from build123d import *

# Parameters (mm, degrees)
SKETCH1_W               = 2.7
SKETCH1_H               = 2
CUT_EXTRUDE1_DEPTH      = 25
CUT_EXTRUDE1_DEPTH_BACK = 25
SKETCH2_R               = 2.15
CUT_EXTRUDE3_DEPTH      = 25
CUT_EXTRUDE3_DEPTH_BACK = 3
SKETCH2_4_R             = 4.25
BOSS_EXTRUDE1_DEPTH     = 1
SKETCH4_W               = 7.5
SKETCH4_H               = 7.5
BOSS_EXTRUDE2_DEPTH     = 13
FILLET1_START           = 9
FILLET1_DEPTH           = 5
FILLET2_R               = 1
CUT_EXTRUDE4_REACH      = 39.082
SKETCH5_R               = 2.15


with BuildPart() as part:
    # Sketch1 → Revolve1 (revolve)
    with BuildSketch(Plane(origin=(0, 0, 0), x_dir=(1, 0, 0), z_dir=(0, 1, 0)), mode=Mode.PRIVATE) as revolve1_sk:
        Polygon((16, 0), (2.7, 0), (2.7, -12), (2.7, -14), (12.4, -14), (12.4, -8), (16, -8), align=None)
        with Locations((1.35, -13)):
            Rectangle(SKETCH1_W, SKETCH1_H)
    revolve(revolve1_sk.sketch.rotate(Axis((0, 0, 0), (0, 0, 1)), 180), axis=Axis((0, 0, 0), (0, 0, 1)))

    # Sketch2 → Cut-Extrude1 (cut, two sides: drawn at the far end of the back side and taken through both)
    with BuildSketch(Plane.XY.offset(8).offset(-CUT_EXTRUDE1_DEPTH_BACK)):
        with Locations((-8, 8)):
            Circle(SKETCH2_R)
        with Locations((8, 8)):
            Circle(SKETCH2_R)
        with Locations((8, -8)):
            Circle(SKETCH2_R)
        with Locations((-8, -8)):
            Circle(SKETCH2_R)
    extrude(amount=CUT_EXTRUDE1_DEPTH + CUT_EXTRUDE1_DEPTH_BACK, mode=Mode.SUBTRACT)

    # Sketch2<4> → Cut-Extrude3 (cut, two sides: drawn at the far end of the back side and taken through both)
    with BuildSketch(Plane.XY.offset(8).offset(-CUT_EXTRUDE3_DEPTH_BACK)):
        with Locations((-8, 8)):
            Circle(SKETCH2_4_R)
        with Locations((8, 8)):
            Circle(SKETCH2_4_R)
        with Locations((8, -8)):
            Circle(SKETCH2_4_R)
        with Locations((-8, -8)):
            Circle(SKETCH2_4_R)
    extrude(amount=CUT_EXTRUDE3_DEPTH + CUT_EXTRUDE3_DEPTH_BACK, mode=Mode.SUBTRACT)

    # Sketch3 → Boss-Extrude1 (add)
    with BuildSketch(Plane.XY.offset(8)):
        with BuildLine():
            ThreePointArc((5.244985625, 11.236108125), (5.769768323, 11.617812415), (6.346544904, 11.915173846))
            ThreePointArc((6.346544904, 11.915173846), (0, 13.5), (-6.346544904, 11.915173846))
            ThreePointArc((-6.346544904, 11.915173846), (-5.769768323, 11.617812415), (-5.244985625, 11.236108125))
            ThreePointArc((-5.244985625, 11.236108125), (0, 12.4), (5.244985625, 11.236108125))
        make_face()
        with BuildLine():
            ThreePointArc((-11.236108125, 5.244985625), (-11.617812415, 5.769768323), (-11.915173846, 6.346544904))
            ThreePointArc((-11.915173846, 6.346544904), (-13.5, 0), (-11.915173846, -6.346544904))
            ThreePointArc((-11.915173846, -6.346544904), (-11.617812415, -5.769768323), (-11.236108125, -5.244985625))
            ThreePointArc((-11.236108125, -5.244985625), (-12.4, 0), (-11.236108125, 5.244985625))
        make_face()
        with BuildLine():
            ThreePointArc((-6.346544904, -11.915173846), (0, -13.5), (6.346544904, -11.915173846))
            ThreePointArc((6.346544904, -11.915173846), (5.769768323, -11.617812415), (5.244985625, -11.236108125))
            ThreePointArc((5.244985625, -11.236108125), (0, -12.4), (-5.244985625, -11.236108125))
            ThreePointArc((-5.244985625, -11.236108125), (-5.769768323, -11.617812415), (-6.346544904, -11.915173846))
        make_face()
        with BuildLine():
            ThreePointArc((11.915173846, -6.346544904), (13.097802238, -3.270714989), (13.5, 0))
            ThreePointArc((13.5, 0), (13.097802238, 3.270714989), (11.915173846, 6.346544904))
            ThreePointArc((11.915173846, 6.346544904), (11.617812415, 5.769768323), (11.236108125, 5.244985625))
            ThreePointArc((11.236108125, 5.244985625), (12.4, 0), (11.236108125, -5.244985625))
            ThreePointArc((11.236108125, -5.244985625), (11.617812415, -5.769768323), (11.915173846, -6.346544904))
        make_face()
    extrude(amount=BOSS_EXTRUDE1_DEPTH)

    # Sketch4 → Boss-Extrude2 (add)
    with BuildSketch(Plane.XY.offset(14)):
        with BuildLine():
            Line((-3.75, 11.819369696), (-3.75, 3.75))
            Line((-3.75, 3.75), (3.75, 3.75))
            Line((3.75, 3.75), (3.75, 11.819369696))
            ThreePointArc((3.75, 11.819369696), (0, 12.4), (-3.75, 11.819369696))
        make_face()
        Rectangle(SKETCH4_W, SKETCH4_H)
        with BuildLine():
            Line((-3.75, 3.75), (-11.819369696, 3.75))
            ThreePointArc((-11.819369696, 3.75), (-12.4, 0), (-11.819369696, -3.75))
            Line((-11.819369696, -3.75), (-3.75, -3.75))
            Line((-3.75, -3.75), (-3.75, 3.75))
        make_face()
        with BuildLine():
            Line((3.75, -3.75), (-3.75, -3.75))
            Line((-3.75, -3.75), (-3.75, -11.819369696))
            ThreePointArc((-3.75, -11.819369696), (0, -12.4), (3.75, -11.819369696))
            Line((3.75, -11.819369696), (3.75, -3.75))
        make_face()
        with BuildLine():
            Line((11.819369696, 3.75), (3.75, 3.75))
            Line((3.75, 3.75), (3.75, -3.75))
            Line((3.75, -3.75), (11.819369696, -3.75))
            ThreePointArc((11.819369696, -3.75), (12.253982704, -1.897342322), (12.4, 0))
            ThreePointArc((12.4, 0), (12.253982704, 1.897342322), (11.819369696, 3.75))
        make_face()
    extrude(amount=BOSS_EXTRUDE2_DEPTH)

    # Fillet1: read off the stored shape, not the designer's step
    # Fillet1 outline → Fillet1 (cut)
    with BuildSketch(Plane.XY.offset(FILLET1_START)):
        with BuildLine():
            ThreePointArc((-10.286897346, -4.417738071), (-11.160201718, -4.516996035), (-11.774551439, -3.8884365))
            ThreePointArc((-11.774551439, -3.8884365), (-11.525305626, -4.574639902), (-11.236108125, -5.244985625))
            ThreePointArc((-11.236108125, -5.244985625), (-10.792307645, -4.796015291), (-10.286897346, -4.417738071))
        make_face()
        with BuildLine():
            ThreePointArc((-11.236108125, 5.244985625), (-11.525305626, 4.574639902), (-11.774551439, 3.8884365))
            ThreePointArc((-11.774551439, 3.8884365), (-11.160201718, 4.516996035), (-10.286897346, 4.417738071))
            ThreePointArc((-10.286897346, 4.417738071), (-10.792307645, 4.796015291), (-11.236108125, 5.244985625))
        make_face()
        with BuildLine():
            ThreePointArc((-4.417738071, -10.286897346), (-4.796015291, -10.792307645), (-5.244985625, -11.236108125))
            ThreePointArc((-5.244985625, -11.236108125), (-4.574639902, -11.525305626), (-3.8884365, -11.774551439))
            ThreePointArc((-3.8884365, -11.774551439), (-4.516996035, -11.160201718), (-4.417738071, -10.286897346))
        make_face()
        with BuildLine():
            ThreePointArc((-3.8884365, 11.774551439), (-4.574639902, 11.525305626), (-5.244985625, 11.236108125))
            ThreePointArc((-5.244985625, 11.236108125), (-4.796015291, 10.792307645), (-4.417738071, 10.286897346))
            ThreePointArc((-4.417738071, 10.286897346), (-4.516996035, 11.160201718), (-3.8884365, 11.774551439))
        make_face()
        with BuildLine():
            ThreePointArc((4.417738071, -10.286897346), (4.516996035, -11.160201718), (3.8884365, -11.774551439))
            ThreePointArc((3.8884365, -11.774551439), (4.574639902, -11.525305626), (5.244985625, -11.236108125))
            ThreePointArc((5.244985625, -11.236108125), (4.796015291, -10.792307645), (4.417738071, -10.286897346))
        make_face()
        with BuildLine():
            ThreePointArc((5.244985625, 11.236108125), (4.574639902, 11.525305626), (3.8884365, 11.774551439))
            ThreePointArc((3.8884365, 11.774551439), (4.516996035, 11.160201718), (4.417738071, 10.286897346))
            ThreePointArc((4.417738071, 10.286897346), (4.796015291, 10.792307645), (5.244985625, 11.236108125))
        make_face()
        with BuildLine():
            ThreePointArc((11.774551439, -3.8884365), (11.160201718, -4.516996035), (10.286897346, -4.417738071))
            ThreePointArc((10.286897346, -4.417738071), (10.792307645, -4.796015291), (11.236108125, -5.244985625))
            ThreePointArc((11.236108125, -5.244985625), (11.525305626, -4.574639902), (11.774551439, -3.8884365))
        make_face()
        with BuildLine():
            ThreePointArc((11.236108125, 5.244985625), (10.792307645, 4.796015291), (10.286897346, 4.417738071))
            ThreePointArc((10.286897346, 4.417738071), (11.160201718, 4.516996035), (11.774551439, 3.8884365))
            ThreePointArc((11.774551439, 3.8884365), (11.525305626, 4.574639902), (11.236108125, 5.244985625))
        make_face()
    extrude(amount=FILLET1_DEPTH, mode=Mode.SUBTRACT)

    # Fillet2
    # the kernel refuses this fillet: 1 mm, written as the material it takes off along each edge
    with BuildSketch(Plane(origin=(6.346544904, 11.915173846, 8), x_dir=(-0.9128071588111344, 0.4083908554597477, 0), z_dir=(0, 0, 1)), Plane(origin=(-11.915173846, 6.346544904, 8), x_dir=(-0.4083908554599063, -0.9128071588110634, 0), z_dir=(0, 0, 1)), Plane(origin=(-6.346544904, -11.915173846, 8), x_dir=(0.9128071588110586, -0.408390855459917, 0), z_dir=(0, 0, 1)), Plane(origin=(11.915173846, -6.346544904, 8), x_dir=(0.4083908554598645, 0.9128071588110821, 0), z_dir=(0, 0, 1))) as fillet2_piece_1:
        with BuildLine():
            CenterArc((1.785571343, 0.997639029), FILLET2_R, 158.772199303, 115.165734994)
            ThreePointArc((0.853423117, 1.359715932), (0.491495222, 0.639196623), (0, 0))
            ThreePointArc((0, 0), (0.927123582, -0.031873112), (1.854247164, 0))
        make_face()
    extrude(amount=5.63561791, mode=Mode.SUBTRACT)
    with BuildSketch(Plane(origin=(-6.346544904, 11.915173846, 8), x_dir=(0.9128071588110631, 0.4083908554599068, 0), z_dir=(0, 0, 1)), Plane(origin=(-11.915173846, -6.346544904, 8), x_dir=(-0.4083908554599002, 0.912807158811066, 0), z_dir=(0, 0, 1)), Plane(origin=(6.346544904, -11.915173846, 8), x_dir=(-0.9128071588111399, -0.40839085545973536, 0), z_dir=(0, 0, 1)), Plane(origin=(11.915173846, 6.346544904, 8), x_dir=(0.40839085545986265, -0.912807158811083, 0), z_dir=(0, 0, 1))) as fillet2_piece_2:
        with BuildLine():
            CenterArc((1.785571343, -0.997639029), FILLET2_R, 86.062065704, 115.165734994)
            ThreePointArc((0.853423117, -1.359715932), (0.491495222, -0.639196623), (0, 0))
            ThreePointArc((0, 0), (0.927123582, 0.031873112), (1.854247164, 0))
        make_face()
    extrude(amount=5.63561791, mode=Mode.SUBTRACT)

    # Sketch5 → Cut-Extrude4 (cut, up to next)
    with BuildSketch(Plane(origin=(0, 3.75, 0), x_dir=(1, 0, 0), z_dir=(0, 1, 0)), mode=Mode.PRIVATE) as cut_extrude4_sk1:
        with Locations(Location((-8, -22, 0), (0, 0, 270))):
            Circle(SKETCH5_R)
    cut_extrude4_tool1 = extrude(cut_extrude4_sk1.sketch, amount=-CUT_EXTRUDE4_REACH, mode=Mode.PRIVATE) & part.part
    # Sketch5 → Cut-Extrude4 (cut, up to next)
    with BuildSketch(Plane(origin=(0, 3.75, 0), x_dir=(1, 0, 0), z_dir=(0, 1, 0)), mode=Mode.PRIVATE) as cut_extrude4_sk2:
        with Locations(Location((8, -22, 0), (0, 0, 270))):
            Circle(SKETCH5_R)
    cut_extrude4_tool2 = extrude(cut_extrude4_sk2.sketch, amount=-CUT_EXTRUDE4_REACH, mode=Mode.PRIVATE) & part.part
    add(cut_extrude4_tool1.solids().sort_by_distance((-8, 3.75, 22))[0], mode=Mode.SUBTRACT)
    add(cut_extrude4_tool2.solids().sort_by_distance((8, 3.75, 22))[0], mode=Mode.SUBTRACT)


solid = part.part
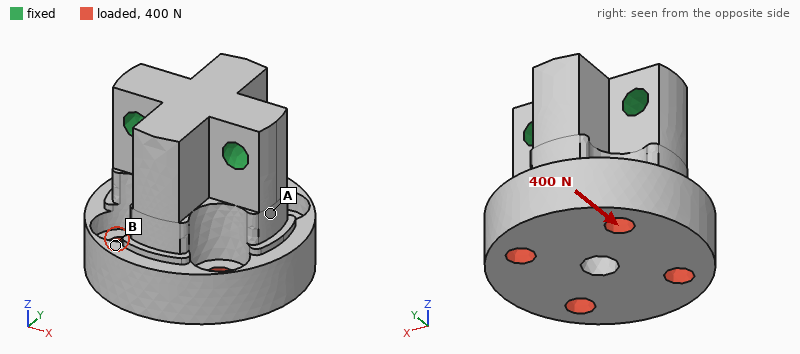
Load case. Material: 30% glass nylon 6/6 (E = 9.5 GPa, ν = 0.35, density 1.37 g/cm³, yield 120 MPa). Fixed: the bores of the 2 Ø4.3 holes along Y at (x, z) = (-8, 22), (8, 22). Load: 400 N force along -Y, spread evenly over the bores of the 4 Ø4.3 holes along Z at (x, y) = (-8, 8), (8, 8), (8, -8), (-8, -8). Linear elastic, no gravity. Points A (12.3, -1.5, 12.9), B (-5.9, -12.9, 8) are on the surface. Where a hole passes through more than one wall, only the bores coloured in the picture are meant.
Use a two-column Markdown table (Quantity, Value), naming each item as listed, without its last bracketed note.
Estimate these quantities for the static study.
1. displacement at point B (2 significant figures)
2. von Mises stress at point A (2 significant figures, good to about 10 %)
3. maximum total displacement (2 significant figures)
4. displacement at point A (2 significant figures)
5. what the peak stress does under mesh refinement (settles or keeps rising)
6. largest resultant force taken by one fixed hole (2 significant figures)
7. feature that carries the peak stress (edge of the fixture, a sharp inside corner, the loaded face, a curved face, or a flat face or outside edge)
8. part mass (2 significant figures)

| Quantity | Value |
|---|---|
| displacement at point B | 0.073 mm |
| von Mises stress at point A | 8.1 MPa |
| maximum total displacement | 0.10 mm |
| displacement at point A | 0.026 mm |
| what the peak stress does under mesh refinement | keeps rising |
| largest resultant force taken by one fixed hole | 200 N |
| feature that carries the peak stress | edge of the fixture |
| part mass | 15 g |
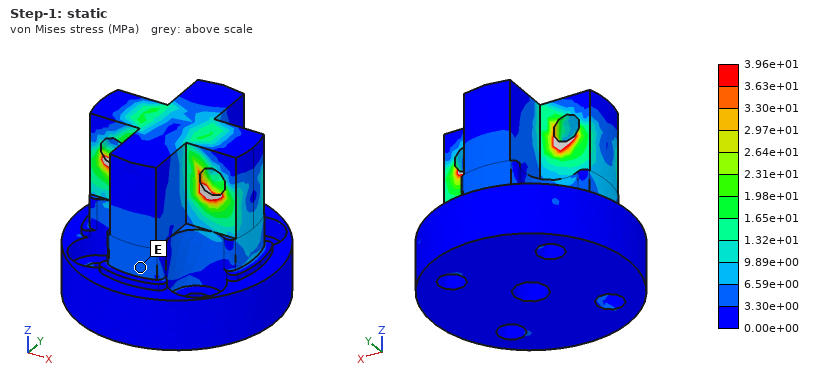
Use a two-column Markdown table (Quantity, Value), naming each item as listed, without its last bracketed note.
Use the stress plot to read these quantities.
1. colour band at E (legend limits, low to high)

| Quantity | Value |
|---|---|
| colour band at E | 3.30e+00 to 6.59e+00 MPa |
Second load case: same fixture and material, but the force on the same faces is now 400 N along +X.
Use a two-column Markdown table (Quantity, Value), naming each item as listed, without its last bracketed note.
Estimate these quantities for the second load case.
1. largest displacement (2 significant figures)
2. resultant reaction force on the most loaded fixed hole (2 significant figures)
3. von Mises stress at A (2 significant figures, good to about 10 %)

| Quantity | Value |
|---|---|
| largest displacement | 27 µm |
| resultant reaction force on the most loaded fixed hole | 470 N |
| von Mises stress at A | 4.7 MPa |
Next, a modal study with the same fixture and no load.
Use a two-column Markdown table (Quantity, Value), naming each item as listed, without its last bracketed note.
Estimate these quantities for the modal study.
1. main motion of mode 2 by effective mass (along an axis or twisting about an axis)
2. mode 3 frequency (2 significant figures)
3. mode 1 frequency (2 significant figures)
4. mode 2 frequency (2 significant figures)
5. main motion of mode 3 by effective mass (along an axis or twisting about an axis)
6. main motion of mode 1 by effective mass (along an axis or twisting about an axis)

| Quantity | Value |
|---|---|
| main motion of mode 2 by effective mass | twisting about Z |
| mode 3 frequency | 7800 Hz |
| mode 1 frequency | 3900 Hz |
| mode 2 frequency | 7000 Hz |
| main motion of mode 3 by effective mass | along X |
| main motion of mode 1 by effective mass | along Y |
